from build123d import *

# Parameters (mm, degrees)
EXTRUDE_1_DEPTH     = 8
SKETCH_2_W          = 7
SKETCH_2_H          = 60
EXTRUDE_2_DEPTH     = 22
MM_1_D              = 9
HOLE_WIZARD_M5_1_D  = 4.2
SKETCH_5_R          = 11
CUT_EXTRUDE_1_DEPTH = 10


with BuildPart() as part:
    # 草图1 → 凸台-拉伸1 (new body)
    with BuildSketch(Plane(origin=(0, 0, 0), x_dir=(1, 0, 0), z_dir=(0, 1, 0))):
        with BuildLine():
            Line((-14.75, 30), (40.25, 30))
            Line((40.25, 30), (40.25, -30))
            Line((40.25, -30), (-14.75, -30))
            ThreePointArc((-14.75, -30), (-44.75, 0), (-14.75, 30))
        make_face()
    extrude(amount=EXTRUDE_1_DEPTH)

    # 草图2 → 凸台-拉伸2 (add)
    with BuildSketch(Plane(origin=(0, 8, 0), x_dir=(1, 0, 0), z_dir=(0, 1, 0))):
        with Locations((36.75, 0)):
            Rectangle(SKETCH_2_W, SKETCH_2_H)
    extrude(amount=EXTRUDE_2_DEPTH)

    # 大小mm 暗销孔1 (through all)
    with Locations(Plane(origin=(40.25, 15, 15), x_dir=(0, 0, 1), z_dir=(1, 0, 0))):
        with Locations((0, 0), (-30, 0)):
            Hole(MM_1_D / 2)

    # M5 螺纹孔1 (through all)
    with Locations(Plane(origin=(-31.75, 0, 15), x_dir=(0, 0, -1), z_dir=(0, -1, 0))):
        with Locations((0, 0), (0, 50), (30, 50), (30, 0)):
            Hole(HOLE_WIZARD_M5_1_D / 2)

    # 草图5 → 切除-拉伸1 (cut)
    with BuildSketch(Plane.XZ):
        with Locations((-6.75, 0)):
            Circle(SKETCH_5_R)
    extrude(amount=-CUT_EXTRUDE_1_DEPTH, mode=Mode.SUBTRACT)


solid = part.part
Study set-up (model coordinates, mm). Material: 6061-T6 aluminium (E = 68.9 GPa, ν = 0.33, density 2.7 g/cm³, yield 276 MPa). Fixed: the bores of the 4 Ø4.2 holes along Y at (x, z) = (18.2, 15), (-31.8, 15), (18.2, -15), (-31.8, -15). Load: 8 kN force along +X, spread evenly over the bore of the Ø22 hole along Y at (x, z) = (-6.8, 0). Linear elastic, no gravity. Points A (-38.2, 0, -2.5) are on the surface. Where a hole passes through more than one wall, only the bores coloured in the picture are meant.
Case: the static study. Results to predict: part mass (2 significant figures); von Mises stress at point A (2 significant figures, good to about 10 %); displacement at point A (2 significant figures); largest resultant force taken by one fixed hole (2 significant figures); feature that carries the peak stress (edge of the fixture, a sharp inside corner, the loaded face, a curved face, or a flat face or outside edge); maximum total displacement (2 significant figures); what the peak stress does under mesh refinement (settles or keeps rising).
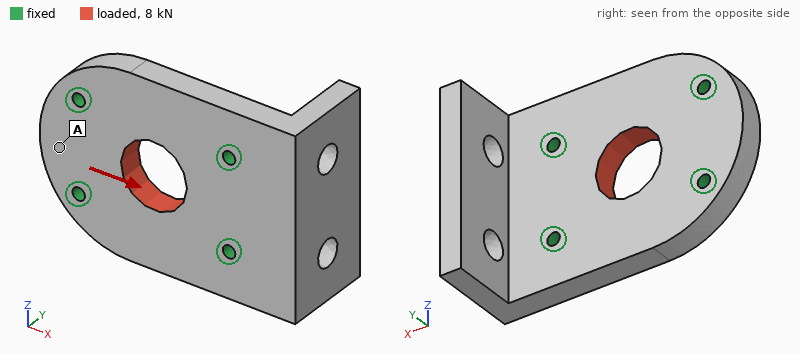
110 g
4.5 MPa
2.5 µm
2.1 kN
edge of the fixture
5.1 µm
keeps rising
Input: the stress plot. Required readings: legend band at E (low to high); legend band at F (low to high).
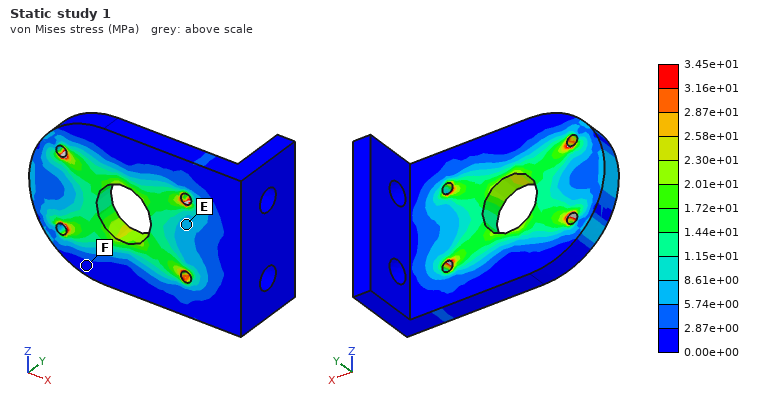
5.74e+00 to 8.61e+00 MPa
0.00e+00 to 2.87e+00 MPa
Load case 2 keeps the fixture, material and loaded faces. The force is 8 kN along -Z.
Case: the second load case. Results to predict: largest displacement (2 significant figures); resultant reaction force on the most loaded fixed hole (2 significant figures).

10 µm
2.2 kN
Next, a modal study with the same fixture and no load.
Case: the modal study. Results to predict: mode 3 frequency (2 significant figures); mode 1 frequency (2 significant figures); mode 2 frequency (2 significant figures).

10000 Hz
4200 Hz
6300 Hz
